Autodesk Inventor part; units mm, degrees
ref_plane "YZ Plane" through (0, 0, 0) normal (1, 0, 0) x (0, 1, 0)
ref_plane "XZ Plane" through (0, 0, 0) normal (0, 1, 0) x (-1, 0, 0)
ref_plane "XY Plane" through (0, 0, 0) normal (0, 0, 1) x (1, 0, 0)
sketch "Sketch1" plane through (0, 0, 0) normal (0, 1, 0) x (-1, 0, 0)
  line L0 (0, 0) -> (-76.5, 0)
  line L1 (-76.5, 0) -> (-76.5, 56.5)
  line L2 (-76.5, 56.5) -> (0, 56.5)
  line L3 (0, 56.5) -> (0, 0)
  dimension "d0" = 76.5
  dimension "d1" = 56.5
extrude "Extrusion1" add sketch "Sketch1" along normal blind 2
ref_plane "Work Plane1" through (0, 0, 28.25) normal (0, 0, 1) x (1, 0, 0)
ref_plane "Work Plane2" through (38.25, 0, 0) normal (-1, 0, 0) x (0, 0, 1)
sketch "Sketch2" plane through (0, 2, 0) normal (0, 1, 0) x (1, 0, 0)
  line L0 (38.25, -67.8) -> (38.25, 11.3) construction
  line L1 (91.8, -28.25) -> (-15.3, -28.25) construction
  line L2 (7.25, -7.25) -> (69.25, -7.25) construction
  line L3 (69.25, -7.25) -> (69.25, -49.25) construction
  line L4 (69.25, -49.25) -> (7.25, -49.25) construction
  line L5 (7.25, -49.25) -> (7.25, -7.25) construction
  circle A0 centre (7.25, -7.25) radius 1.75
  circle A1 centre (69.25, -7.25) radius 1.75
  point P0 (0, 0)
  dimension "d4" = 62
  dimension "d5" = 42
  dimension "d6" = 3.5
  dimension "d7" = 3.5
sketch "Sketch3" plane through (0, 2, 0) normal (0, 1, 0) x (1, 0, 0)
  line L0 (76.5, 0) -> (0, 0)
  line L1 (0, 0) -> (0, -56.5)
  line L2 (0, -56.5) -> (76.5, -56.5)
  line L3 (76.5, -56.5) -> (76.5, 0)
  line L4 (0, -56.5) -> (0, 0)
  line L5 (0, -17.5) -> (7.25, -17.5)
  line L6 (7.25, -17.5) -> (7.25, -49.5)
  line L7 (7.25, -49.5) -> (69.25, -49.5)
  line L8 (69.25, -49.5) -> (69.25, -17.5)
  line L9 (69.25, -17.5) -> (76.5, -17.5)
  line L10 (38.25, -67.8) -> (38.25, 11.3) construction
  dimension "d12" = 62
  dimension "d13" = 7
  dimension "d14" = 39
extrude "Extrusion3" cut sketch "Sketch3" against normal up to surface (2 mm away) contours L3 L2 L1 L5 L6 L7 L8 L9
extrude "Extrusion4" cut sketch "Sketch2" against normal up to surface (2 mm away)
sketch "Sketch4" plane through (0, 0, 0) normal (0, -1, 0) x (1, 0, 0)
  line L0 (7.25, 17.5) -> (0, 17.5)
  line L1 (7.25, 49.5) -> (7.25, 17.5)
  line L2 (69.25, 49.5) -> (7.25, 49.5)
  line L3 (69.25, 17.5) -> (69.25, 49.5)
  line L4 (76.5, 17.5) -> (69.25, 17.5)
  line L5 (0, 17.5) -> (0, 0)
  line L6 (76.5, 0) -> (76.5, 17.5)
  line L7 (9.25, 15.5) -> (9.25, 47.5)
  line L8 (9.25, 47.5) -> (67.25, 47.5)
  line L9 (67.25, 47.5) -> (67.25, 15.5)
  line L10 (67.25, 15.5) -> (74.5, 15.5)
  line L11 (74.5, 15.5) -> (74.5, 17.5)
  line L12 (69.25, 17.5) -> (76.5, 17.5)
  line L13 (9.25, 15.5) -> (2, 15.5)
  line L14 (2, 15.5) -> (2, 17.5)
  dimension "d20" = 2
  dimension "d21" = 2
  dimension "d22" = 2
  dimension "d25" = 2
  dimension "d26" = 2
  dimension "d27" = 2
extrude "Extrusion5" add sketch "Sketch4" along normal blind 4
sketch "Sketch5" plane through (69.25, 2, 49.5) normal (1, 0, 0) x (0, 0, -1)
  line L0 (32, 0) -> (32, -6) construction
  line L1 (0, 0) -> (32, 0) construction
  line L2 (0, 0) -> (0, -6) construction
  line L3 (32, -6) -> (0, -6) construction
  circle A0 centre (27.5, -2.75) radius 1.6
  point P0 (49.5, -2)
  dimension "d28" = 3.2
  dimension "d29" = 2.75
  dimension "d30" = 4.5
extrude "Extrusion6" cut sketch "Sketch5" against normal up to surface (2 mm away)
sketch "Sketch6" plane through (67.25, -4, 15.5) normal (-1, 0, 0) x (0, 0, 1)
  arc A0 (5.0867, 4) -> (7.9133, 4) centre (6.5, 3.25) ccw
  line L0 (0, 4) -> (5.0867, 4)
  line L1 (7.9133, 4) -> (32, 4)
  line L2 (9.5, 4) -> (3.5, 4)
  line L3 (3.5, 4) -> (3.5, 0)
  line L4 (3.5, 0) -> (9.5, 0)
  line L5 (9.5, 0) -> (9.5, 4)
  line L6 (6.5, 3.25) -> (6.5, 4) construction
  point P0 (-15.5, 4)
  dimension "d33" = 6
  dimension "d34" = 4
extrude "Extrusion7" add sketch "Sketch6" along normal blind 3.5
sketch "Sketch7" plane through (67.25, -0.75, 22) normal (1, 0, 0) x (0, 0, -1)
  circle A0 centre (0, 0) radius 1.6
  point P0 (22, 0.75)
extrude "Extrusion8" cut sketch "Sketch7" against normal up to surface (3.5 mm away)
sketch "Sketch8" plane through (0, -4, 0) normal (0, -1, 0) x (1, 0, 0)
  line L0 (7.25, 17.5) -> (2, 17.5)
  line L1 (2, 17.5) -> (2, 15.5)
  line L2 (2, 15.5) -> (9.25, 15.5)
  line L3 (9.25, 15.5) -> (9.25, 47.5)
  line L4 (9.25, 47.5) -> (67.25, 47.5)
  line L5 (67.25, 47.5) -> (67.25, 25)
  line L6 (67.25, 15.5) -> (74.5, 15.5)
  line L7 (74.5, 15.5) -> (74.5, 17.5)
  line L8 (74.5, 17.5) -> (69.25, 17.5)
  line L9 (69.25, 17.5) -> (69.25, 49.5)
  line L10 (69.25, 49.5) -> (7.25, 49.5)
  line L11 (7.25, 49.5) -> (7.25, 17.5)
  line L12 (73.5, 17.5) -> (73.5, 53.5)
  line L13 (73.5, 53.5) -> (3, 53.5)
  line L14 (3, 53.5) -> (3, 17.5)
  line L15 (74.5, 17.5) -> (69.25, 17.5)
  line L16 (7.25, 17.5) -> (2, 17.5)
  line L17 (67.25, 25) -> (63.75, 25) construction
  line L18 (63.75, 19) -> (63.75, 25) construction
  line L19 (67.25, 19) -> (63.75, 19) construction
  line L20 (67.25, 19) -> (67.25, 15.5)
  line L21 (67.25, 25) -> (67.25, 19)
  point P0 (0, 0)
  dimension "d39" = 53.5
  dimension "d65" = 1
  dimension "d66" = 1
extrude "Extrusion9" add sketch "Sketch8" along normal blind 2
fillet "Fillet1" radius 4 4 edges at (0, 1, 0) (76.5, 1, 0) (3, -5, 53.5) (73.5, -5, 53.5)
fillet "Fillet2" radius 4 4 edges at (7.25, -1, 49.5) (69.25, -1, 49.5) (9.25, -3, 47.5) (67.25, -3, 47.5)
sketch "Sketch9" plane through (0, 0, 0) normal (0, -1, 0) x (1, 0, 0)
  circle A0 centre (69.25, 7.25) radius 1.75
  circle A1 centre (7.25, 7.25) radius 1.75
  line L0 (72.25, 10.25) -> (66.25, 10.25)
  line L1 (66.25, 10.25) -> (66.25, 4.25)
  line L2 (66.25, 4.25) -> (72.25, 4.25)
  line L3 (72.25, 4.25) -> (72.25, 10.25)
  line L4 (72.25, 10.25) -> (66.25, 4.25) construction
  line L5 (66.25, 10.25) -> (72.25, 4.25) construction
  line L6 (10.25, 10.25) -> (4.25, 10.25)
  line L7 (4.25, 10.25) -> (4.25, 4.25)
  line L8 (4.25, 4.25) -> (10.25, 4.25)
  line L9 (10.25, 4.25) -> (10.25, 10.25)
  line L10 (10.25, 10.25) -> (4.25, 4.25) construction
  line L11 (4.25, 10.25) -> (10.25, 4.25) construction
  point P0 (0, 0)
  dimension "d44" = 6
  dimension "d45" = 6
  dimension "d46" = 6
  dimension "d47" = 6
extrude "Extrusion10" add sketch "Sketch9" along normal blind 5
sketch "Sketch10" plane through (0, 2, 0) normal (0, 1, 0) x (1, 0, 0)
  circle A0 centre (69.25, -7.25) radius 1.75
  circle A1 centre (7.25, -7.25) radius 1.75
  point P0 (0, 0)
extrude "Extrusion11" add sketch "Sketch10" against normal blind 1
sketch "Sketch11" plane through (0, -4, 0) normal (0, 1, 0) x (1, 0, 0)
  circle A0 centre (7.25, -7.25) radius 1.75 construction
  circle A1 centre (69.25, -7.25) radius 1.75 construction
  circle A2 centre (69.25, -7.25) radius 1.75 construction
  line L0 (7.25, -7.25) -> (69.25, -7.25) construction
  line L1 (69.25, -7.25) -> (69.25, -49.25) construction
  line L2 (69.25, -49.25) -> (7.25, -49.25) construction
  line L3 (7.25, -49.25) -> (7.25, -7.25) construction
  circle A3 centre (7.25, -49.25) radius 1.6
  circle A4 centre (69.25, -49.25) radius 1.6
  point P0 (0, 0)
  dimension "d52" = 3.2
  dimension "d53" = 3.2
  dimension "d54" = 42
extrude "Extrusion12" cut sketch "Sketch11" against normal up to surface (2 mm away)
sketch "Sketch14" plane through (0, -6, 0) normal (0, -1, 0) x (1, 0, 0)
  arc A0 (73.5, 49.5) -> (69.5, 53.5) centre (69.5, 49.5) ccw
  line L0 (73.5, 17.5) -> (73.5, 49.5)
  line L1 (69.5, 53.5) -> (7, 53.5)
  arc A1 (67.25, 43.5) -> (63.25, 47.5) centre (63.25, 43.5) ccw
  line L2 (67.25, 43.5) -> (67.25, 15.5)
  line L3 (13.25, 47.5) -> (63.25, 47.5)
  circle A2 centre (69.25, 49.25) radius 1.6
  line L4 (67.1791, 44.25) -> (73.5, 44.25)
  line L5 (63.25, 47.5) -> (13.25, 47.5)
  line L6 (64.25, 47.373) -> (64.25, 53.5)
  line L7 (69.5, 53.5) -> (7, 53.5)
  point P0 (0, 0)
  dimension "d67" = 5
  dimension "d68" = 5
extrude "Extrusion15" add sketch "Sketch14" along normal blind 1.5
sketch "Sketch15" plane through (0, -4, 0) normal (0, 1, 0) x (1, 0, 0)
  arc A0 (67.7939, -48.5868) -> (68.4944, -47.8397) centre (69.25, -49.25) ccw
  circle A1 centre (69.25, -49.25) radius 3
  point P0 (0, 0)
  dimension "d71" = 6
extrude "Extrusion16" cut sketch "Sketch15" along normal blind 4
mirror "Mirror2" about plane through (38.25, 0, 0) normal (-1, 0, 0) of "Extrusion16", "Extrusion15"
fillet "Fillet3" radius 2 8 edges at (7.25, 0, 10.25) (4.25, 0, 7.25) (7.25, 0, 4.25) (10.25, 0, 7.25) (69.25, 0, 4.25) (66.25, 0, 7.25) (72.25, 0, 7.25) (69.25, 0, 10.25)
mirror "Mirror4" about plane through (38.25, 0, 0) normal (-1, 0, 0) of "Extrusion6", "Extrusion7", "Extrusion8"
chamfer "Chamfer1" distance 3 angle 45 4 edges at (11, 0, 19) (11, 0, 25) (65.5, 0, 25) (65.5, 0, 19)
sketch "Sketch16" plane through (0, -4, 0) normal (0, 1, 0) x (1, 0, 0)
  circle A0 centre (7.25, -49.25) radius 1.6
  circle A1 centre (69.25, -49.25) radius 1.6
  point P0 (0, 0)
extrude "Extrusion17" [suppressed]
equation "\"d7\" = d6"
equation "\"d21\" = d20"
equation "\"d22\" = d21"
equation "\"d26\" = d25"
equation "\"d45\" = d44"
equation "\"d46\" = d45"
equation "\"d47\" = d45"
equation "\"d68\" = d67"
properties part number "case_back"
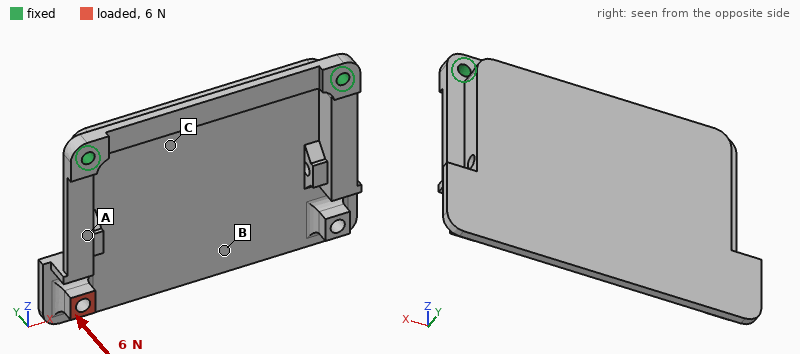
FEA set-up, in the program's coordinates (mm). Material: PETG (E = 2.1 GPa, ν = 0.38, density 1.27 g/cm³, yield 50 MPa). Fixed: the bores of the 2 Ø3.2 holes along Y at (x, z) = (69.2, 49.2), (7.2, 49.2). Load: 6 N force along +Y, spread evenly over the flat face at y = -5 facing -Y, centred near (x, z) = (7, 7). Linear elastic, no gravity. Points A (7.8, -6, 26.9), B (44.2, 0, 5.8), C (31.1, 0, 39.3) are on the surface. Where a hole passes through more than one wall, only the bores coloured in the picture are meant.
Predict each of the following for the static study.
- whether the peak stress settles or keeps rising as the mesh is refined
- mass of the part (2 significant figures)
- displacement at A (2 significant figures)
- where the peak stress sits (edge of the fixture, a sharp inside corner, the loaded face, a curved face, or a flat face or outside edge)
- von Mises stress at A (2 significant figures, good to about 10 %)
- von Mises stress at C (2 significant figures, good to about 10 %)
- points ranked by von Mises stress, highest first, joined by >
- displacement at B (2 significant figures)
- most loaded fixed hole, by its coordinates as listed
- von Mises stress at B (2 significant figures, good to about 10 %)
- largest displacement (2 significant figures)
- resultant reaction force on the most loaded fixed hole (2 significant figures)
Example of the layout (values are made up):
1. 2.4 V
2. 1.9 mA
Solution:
1. keeps rising
2. 13 g
3. 0.32 mm
4. edge of the fixture
5. 2.0 MPa
6. 0.56 MPa
7. A > B > C
8. 0.38 mm
9. (7.2, 49.2)
10. 0.99 MPa
11. 0.97 mm
12. 7.0 N
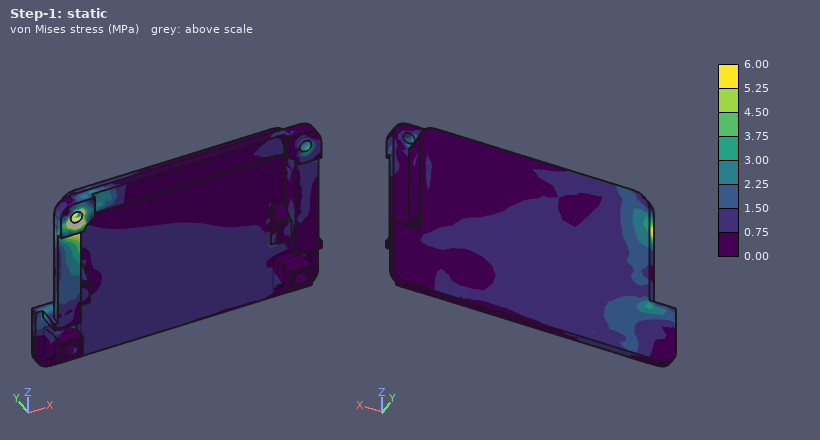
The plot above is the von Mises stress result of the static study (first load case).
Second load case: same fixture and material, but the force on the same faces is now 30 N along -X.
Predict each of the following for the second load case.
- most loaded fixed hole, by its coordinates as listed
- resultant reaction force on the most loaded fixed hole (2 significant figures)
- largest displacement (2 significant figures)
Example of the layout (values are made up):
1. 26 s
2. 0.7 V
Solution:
1. (7.2, 49.2)
2. 30 N
3. 0.88 mm
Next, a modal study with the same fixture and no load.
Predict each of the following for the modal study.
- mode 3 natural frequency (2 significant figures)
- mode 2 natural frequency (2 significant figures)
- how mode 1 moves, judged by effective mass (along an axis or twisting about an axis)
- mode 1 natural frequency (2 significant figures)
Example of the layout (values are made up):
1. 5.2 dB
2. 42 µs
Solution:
1. 790 Hz
2. 410 Hz
3. along Y
4. 260 Hz
